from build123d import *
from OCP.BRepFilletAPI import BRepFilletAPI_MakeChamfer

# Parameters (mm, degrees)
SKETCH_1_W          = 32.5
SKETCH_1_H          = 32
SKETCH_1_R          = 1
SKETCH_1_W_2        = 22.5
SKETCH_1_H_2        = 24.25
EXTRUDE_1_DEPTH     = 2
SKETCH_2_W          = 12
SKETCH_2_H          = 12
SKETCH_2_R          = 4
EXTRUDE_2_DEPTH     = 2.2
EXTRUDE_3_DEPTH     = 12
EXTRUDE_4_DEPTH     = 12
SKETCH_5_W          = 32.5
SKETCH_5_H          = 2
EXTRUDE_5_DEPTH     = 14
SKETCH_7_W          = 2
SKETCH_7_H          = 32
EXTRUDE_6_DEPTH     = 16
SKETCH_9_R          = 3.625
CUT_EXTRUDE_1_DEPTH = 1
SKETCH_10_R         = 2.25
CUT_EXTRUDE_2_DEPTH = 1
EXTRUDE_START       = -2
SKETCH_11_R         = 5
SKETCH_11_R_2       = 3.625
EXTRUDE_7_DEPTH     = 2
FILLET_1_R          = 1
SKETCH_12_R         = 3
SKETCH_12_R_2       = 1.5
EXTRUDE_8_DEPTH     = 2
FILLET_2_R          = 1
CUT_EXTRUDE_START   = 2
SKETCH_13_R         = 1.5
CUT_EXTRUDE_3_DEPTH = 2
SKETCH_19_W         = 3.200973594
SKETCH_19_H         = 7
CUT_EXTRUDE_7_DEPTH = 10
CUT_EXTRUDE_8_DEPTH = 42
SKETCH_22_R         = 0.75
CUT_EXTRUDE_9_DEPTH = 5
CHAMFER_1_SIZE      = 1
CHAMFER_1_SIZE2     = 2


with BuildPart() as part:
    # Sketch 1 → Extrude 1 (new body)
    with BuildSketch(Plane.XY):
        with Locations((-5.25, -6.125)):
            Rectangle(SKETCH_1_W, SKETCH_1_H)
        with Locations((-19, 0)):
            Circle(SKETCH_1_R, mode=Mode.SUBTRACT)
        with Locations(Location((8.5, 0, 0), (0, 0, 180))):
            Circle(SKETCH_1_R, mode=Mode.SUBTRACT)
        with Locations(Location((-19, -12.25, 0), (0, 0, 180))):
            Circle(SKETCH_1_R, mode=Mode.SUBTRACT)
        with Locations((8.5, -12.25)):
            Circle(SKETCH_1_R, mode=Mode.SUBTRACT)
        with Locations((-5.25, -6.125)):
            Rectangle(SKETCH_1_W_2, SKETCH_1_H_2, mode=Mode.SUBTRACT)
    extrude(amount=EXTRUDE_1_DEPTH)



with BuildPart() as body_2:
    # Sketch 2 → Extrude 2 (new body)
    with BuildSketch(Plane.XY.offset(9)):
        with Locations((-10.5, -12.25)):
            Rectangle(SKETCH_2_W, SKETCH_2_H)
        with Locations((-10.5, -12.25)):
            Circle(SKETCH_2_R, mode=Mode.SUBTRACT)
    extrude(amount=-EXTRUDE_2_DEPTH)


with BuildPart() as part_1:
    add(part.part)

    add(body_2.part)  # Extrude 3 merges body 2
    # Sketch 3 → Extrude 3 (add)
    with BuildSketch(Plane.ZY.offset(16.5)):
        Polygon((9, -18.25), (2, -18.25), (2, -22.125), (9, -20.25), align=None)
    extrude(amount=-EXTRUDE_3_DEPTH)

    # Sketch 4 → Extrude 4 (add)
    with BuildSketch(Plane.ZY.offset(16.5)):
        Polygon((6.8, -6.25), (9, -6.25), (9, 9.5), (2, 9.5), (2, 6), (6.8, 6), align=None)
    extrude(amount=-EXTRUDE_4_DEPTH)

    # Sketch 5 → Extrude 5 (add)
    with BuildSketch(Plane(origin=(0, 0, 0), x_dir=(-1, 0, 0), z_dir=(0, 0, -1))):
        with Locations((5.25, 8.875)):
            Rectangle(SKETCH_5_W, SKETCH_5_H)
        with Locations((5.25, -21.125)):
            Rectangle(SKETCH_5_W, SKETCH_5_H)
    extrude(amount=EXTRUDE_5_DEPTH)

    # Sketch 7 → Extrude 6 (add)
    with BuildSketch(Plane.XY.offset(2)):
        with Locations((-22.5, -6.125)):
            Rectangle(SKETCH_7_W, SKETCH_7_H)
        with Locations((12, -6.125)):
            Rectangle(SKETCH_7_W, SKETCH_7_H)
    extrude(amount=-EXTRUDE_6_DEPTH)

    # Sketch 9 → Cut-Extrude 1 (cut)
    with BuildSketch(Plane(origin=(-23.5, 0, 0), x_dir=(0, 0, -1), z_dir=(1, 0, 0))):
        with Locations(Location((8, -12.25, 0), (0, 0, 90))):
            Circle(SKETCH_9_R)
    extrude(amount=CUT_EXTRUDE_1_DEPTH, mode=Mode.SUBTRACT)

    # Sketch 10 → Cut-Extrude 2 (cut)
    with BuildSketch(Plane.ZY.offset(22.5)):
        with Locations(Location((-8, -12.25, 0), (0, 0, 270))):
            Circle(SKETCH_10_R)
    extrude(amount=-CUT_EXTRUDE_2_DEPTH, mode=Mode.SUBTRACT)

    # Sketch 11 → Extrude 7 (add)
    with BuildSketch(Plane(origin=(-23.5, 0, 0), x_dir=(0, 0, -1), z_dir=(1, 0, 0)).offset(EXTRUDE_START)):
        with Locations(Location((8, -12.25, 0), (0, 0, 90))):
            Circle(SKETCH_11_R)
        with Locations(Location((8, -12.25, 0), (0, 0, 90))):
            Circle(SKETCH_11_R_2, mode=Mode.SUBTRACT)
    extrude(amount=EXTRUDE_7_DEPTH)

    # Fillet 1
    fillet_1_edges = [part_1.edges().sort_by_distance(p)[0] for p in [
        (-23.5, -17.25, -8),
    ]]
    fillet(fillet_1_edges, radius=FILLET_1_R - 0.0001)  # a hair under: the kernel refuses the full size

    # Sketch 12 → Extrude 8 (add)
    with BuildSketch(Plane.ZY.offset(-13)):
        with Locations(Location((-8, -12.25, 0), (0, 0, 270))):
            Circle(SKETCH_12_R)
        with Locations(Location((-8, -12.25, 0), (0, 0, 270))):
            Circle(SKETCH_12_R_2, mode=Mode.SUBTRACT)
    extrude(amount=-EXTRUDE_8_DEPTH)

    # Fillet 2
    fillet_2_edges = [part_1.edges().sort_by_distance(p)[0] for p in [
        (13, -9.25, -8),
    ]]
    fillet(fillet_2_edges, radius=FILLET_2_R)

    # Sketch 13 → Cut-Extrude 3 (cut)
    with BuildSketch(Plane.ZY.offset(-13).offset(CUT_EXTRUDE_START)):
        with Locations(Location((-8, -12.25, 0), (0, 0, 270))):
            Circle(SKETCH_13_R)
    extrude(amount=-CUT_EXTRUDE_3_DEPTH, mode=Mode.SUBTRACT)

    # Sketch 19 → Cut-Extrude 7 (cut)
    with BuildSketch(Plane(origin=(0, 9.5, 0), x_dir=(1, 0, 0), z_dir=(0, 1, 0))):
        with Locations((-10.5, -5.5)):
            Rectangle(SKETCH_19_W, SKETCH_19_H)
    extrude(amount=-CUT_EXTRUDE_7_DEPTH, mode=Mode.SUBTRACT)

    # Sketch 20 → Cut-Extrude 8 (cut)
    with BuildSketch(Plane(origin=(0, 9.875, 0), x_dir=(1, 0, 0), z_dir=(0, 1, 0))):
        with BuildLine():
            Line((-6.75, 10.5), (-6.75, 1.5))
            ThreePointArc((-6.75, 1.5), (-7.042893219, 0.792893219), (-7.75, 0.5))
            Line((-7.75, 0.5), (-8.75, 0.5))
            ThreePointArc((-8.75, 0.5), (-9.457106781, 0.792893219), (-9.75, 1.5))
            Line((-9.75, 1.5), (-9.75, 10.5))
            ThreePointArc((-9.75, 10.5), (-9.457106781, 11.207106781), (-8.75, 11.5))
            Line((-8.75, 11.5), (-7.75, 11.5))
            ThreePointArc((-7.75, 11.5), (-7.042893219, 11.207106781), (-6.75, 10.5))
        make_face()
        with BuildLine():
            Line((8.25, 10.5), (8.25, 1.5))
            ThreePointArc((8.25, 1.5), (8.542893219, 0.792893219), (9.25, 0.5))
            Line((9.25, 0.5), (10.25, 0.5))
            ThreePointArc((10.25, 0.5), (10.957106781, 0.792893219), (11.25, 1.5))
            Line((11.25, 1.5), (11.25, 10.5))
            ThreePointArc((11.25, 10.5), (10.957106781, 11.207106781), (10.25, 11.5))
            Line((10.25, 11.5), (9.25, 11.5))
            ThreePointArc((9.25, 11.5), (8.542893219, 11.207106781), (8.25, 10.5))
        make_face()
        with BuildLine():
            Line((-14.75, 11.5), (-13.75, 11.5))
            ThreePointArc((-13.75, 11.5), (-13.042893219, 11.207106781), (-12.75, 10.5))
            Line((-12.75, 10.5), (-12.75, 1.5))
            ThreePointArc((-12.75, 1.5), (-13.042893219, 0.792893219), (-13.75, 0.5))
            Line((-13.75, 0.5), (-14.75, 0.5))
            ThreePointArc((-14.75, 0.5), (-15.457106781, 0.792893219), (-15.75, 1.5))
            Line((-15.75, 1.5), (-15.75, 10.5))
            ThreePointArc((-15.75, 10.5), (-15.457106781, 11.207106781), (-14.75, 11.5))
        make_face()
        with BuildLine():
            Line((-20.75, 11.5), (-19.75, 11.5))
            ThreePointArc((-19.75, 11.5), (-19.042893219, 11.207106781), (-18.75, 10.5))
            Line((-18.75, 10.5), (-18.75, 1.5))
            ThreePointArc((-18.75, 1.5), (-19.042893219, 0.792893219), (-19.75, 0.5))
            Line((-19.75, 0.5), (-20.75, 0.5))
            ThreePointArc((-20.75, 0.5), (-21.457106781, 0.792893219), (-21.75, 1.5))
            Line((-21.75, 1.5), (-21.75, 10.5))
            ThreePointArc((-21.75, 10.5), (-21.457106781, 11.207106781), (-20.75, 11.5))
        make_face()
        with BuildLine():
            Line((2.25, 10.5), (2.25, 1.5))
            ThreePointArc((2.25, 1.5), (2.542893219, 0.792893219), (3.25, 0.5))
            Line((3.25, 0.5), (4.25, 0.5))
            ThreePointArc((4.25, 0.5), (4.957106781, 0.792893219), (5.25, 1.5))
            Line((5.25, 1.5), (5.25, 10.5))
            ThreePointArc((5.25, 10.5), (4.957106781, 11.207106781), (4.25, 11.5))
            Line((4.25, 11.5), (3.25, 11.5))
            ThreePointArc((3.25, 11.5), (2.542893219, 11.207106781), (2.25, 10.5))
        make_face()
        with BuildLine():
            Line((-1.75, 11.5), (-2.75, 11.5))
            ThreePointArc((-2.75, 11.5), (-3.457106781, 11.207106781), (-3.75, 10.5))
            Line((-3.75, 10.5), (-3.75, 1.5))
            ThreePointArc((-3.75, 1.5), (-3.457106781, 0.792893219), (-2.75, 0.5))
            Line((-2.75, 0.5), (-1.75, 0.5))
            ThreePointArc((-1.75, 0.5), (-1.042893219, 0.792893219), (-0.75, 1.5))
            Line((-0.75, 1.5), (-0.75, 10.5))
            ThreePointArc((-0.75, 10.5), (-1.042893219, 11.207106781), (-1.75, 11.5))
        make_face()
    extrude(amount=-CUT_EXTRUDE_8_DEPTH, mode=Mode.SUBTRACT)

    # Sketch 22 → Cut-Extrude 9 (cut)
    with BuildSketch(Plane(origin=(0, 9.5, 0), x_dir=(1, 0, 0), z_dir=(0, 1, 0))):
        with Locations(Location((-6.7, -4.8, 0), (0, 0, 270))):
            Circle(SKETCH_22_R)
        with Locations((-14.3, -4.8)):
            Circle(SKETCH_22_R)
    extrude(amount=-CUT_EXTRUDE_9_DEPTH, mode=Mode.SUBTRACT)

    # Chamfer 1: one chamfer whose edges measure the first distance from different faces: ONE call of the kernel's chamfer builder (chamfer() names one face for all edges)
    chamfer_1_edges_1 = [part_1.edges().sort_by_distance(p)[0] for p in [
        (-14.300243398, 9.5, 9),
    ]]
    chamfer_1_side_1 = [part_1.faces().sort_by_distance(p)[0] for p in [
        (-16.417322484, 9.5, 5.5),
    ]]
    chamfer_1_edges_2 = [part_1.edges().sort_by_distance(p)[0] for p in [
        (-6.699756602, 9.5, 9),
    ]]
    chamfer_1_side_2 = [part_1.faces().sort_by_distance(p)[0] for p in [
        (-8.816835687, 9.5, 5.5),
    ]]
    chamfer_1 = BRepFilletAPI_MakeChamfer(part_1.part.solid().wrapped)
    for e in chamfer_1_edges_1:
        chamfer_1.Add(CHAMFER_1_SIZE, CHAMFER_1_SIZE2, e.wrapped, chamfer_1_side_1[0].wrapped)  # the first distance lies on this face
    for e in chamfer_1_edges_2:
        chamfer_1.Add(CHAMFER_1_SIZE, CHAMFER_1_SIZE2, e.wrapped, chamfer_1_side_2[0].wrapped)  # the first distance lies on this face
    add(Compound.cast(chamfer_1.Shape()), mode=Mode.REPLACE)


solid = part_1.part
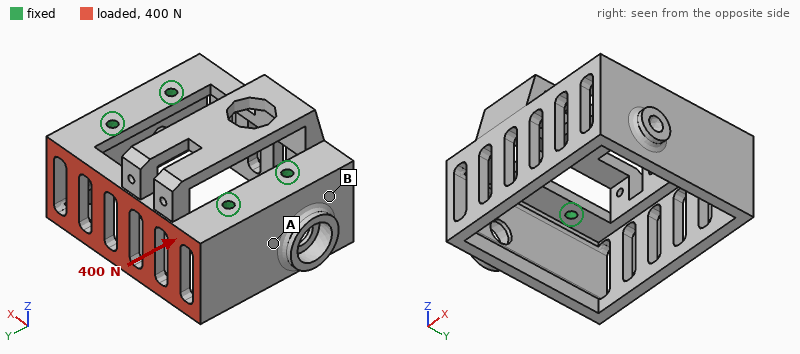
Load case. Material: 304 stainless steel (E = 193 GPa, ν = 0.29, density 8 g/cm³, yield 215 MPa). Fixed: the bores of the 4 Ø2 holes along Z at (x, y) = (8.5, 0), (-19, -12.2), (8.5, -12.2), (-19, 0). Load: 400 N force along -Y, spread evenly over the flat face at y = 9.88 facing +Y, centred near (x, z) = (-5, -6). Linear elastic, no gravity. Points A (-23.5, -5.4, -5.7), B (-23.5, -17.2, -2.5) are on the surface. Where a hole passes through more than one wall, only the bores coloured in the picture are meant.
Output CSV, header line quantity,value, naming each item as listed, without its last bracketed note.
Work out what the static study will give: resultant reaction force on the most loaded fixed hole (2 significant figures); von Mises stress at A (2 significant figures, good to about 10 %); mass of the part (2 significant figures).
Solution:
quantity,value
resultant reaction force on the most loaded fixed hole,230 N
von Mises stress at A,14 MPa
mass of the part,39 g
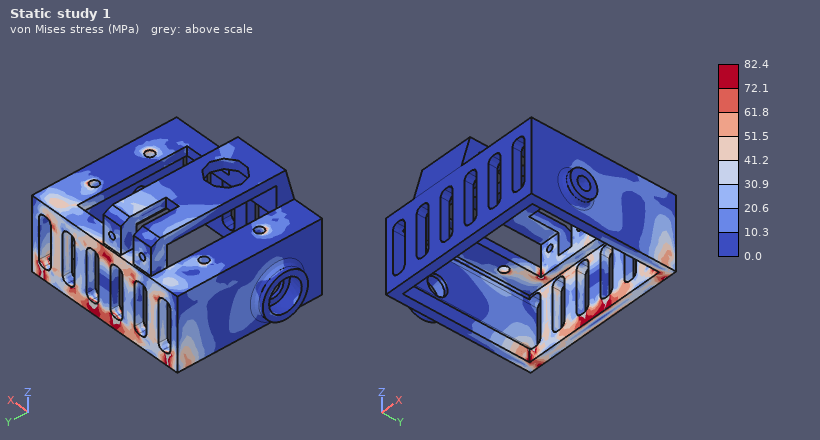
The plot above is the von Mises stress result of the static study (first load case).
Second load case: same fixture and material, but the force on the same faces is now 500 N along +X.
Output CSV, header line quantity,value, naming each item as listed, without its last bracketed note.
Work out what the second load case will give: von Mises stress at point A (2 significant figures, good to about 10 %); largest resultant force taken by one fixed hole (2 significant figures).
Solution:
quantity,value
von Mises stress at point A,12 MPa
largest resultant force taken by one fixed hole,350 N
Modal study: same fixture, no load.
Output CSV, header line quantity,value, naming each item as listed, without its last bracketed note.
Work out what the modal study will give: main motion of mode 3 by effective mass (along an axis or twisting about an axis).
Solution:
quantity,value
main motion of mode 3 by effective mass,along X
